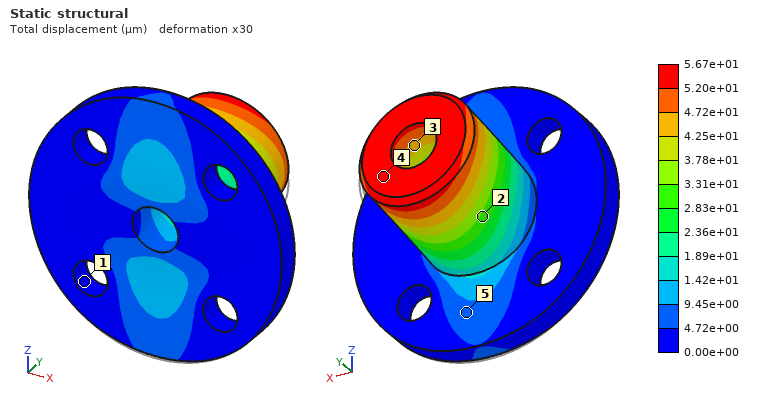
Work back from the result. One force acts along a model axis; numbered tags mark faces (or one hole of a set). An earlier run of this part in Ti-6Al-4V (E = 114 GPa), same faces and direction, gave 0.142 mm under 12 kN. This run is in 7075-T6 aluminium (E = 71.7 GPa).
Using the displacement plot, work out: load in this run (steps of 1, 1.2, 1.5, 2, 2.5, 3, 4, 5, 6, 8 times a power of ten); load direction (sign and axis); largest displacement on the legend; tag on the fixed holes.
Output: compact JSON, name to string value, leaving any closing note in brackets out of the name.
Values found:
{"load in this run": "3 kN", "load direction": "+Z", "largest displacement on the legend": "5.67e+01 µm", "tag on the fixed holes": "1"}
